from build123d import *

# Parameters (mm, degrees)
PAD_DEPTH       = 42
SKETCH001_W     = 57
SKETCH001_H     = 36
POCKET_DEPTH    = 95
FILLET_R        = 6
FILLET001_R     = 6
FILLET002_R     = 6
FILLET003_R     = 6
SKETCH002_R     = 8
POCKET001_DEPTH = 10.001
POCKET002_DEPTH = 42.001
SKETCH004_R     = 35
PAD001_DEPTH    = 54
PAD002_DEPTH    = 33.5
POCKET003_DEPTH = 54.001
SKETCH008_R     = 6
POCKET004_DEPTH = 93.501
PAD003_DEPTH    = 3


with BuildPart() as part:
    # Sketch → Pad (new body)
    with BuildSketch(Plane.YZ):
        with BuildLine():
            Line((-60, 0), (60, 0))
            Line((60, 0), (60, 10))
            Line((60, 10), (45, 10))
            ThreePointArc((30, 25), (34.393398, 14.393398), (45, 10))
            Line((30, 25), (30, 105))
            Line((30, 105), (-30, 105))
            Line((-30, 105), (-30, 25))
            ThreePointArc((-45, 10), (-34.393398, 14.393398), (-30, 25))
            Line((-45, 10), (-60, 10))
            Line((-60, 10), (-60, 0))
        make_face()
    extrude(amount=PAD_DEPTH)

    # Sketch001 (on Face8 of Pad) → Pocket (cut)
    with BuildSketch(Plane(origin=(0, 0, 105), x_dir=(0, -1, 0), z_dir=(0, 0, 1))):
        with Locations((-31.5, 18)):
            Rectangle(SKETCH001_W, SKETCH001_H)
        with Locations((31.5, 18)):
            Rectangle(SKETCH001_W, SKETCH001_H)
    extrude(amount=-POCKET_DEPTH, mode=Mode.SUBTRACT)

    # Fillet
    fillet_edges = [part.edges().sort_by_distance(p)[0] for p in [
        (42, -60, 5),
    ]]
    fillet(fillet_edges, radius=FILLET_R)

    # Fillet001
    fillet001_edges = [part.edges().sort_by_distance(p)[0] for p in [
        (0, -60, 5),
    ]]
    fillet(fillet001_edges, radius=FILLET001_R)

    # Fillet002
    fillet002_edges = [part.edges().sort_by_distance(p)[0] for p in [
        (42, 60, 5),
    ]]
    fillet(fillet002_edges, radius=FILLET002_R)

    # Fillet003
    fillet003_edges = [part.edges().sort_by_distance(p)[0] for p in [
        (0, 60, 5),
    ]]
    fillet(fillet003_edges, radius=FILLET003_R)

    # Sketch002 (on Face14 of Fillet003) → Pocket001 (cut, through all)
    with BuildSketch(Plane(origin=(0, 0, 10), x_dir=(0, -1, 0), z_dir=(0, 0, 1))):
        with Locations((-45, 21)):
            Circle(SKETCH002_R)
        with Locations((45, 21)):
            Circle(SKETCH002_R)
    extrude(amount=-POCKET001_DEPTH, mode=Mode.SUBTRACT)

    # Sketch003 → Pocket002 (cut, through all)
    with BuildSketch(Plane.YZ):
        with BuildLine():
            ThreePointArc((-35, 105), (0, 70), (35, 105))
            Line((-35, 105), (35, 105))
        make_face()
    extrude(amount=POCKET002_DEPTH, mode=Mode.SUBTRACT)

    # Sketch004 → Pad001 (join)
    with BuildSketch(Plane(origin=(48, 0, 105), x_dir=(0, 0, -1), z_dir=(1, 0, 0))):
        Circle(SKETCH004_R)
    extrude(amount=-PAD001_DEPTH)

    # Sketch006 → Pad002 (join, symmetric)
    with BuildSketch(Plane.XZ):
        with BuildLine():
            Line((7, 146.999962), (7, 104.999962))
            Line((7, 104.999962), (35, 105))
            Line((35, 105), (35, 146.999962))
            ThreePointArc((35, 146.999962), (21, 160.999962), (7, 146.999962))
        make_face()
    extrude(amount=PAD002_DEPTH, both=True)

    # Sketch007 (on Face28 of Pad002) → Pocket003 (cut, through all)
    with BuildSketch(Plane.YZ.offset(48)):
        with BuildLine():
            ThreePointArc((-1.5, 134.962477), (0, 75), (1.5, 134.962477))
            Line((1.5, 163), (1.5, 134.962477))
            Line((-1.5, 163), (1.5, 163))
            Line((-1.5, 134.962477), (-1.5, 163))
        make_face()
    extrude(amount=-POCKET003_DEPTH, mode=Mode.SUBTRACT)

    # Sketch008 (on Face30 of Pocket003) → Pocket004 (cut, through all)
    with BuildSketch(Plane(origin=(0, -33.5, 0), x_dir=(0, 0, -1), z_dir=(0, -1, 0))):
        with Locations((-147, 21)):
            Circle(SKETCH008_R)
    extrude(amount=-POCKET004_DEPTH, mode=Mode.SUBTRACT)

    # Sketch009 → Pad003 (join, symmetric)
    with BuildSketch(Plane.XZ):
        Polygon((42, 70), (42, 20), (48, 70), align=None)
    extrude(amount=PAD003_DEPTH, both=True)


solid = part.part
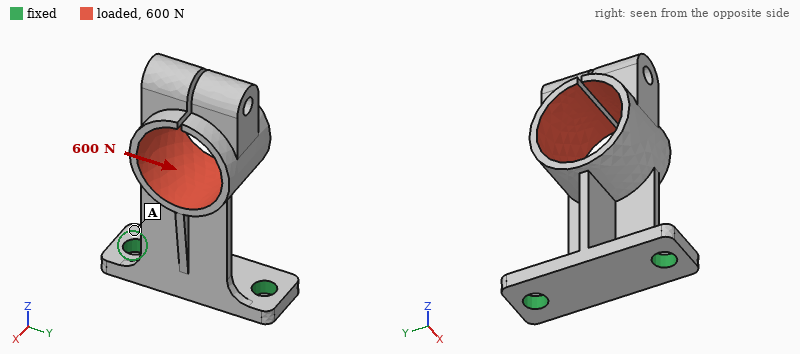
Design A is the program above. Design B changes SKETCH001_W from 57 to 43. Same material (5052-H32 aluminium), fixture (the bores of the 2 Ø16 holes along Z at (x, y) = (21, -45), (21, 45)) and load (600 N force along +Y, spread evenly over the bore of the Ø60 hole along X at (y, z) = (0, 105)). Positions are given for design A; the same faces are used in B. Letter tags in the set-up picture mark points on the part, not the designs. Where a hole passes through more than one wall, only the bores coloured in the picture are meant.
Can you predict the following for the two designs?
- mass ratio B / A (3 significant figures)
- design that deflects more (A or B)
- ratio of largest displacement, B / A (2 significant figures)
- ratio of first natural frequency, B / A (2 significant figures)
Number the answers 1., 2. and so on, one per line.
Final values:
1. 1.17
2. A
3. 0.83
4. 1.1
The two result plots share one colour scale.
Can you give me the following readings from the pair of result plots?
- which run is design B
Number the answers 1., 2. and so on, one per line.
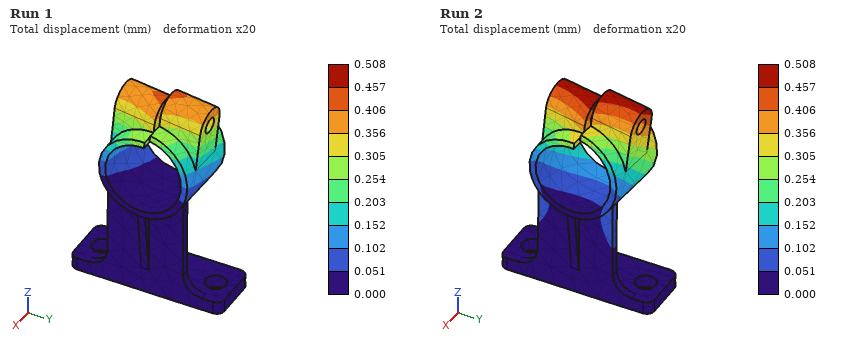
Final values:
1. Run 1
